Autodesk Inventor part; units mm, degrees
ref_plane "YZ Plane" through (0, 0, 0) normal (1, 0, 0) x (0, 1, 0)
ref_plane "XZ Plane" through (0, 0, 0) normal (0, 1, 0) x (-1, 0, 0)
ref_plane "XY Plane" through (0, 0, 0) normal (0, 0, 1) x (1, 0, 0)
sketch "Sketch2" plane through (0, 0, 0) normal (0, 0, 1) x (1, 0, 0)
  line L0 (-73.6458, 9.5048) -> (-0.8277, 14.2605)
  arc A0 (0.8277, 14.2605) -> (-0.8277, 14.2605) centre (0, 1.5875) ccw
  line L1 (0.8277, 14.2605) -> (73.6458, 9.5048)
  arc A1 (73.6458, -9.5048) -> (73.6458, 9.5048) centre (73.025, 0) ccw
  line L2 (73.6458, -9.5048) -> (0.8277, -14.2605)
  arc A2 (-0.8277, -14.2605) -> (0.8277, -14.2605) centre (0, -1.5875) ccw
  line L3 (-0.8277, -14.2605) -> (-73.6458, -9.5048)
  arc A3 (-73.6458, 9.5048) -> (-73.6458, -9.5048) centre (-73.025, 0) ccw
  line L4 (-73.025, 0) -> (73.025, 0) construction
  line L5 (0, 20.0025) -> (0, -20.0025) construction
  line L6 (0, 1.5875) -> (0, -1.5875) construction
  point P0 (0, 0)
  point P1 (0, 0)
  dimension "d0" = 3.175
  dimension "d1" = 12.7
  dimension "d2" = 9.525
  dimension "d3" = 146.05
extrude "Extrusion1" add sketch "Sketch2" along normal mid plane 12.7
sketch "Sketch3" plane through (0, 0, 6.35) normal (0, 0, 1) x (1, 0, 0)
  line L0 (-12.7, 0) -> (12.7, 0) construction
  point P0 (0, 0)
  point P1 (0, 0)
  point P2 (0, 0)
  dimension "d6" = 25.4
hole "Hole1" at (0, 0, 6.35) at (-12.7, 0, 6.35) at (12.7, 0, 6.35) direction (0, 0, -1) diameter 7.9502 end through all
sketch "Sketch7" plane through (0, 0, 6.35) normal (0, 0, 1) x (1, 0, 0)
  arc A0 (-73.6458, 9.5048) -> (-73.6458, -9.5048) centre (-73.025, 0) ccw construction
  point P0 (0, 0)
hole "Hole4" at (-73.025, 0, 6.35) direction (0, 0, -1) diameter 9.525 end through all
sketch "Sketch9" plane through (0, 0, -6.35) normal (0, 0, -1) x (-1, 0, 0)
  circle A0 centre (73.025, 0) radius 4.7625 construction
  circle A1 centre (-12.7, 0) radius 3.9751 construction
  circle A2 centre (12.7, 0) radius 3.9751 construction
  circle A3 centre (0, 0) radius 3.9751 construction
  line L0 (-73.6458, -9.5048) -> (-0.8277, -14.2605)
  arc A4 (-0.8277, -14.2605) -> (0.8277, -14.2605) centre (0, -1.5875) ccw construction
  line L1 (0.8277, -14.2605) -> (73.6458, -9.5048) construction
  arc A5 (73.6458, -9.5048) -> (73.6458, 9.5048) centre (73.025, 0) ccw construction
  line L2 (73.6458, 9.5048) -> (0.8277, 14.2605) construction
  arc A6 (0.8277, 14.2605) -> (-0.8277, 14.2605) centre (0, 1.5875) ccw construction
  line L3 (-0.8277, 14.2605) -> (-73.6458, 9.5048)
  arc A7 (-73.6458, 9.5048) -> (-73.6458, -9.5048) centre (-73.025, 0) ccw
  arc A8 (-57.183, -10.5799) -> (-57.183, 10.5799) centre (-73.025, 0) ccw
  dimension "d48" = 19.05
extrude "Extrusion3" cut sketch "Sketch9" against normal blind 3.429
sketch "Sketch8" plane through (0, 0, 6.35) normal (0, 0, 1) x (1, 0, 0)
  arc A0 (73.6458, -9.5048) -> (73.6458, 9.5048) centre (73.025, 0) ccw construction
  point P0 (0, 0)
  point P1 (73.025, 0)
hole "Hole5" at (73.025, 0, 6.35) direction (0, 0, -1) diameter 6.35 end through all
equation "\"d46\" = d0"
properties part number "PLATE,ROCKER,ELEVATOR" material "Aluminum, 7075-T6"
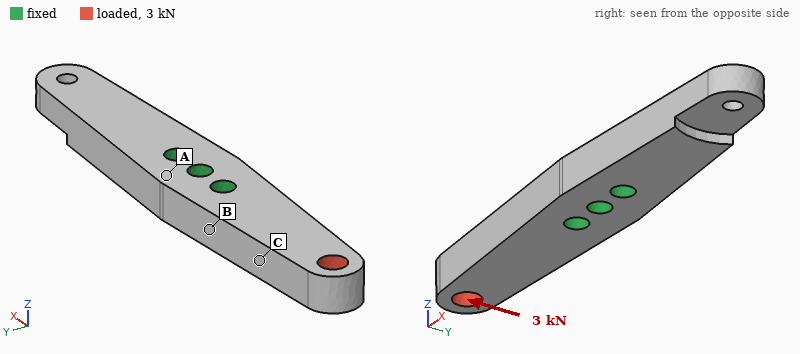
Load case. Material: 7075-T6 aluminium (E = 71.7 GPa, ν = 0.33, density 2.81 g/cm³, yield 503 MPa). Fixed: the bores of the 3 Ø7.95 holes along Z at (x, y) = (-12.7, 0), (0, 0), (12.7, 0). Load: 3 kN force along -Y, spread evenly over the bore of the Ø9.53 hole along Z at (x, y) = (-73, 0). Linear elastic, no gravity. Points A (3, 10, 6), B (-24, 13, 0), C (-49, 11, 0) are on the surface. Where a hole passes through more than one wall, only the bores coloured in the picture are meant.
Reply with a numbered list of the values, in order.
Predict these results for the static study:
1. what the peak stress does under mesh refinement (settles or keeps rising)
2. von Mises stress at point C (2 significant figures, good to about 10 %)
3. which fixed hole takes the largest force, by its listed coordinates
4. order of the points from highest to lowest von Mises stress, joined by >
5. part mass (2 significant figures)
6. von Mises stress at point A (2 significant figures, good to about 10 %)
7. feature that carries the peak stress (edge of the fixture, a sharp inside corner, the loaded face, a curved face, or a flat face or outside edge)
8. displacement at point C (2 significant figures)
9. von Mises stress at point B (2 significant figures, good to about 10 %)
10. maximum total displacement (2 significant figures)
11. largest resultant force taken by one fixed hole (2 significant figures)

1. keeps rising
2. 69 MPa
3. (-12.7, 0)
4. B > C > A
5. 120 g
6. 19 MPa
7. edge of the fixture
8. 0.14 mm
9. 110 MPa
10. 0.33 mm
11. 7.8 kN
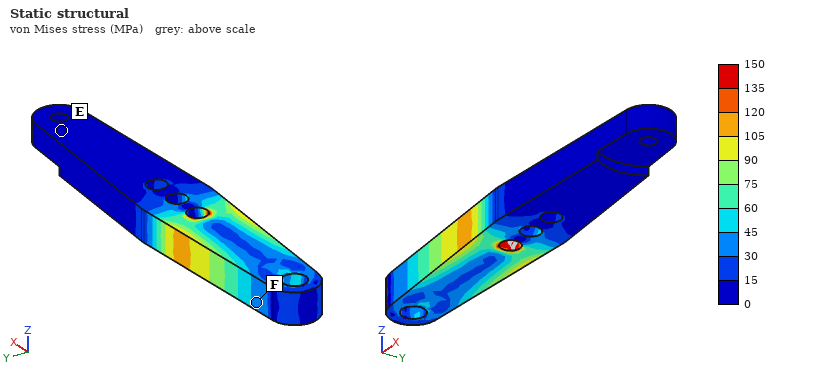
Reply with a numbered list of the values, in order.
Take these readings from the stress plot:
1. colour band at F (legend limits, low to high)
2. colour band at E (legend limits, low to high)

1. 30 to 45 MPa
2. 0 to 15 MPa
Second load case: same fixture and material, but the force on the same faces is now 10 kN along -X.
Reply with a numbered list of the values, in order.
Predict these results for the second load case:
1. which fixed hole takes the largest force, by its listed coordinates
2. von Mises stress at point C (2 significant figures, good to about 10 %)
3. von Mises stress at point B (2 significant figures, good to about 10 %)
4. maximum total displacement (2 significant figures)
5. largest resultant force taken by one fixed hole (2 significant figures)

1. (-12.7, 0)
2. 36 MPa
3. 22 MPa
4. 42 µm
5. 8.1 kN
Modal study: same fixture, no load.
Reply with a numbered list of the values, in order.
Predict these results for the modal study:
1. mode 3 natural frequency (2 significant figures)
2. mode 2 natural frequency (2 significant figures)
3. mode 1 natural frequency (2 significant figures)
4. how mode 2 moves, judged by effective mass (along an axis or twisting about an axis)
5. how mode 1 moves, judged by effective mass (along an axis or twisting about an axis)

1. 4300 Hz
2. 2900 Hz
3. 2700 Hz
4. along Z
5. along Z
